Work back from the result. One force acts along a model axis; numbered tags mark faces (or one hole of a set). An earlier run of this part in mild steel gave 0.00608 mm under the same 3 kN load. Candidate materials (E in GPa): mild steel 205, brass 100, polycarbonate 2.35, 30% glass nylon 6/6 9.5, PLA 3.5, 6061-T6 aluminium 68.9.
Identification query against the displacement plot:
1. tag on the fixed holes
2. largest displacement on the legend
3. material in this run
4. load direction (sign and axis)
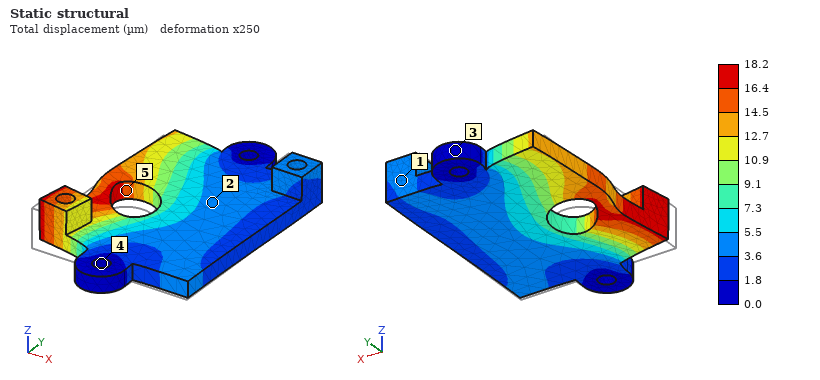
4
18.2 µm
6061-T6 aluminium
+Y
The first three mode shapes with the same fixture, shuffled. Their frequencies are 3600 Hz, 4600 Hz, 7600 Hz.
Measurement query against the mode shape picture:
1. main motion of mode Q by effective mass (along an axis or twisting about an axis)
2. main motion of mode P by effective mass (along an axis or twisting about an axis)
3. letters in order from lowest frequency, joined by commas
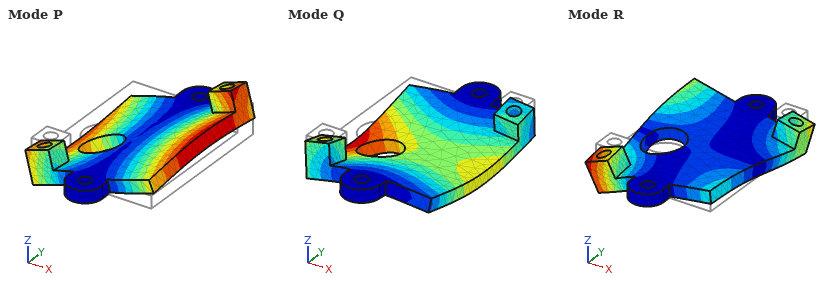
along Z
twisting about Y
P, Q, R
